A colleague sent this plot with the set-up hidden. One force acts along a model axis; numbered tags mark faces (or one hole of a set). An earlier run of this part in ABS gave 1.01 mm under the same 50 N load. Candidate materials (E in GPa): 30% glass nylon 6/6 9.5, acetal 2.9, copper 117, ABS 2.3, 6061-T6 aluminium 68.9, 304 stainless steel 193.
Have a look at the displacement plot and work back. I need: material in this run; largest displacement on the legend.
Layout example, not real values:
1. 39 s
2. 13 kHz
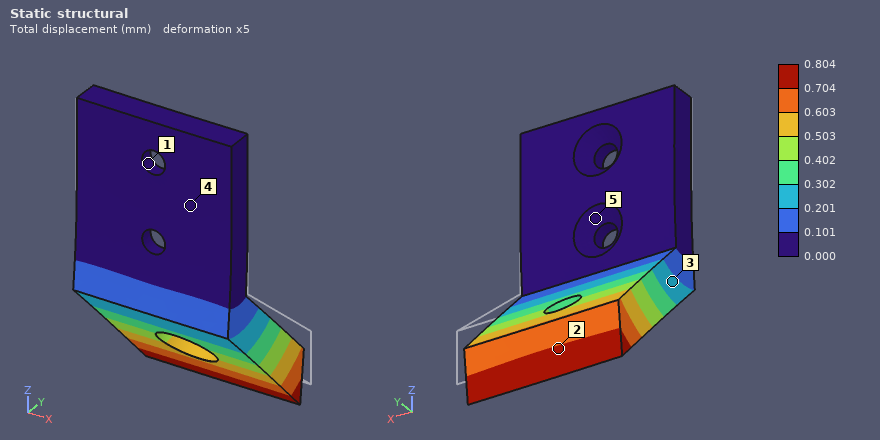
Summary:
1. acetal
2. 0.804 mm
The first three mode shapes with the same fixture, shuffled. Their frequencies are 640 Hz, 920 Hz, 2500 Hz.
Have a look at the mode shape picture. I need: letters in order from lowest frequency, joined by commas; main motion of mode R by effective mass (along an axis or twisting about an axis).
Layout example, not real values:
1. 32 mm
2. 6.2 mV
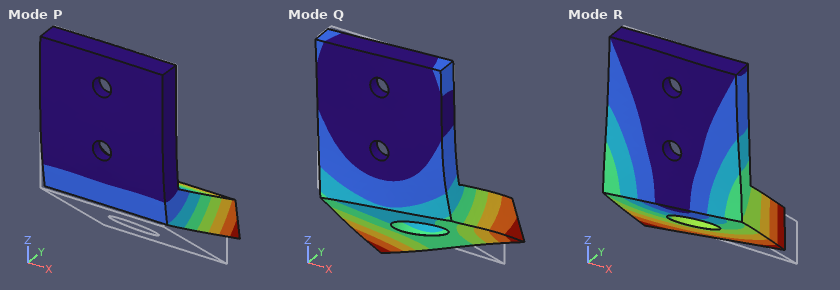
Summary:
1. P, R, Q
2. along X
